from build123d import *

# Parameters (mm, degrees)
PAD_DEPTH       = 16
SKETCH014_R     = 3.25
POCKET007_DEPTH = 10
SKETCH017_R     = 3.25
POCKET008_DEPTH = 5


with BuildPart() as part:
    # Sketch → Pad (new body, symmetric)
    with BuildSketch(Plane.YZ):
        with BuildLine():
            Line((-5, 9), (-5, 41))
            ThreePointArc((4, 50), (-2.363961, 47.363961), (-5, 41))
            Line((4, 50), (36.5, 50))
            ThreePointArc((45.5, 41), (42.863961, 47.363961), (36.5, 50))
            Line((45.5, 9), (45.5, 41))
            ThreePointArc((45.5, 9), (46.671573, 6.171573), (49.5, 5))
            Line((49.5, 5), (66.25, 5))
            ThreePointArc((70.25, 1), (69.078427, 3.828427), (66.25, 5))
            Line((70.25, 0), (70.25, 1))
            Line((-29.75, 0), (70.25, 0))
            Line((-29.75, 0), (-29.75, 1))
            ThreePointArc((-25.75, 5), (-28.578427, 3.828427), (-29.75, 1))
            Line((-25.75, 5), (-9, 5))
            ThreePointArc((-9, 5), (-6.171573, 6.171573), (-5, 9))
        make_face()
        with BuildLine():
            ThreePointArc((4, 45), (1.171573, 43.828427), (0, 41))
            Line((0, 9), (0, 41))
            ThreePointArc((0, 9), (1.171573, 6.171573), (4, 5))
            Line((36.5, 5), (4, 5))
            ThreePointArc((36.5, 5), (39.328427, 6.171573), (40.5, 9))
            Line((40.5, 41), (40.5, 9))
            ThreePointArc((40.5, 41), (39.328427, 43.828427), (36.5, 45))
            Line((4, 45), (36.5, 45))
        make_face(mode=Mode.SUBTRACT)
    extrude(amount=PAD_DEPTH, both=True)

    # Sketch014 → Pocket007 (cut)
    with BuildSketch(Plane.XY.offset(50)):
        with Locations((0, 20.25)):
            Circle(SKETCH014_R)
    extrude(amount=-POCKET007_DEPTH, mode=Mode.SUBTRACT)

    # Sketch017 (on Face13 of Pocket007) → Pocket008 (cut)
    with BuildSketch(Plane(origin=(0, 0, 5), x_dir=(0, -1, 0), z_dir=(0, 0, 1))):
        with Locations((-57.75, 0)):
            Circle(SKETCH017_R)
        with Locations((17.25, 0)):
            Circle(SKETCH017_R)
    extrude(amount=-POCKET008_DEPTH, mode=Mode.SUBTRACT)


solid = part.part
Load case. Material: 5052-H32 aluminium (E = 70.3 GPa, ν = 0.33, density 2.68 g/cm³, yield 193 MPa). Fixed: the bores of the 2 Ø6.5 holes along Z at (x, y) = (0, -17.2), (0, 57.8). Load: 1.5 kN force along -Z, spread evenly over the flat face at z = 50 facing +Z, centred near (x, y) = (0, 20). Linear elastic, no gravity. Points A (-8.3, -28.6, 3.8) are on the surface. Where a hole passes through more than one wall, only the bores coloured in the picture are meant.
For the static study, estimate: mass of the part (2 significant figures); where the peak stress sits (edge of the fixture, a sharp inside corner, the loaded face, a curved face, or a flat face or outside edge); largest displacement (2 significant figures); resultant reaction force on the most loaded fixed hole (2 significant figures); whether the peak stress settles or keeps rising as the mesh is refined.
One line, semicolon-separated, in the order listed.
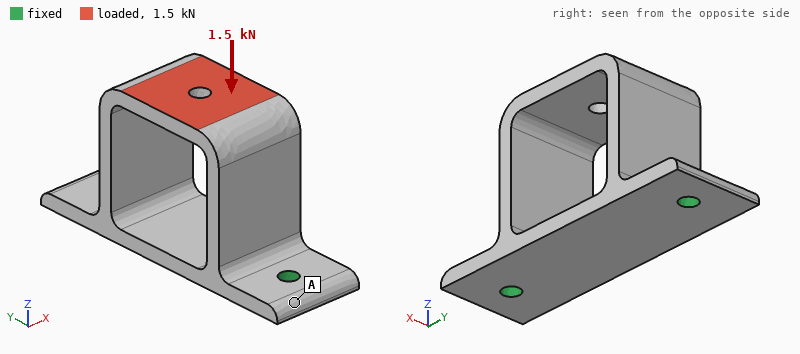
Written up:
96 g; edge of the fixture; 56 µm; 780 N; keeps rising
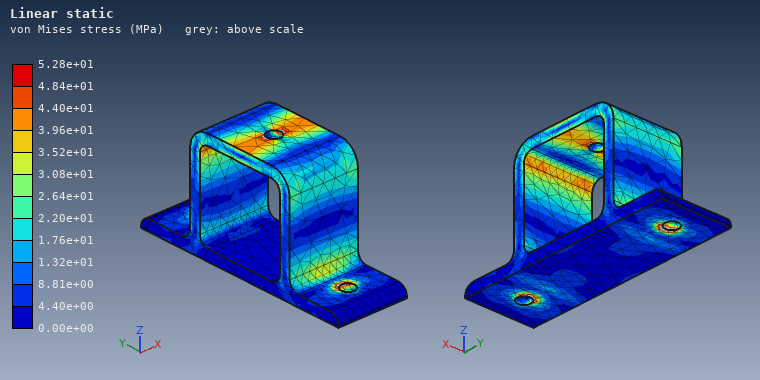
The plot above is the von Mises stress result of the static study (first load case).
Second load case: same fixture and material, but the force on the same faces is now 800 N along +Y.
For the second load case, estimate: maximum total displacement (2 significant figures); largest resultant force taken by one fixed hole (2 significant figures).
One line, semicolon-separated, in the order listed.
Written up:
0.15 mm; 690 N
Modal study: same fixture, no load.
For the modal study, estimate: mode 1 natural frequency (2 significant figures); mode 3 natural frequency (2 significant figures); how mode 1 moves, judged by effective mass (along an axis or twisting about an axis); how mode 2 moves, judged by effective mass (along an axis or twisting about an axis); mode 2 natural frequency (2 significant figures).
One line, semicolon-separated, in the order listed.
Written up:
1700 Hz; 3600 Hz; along X; along Y; 2200 Hz
